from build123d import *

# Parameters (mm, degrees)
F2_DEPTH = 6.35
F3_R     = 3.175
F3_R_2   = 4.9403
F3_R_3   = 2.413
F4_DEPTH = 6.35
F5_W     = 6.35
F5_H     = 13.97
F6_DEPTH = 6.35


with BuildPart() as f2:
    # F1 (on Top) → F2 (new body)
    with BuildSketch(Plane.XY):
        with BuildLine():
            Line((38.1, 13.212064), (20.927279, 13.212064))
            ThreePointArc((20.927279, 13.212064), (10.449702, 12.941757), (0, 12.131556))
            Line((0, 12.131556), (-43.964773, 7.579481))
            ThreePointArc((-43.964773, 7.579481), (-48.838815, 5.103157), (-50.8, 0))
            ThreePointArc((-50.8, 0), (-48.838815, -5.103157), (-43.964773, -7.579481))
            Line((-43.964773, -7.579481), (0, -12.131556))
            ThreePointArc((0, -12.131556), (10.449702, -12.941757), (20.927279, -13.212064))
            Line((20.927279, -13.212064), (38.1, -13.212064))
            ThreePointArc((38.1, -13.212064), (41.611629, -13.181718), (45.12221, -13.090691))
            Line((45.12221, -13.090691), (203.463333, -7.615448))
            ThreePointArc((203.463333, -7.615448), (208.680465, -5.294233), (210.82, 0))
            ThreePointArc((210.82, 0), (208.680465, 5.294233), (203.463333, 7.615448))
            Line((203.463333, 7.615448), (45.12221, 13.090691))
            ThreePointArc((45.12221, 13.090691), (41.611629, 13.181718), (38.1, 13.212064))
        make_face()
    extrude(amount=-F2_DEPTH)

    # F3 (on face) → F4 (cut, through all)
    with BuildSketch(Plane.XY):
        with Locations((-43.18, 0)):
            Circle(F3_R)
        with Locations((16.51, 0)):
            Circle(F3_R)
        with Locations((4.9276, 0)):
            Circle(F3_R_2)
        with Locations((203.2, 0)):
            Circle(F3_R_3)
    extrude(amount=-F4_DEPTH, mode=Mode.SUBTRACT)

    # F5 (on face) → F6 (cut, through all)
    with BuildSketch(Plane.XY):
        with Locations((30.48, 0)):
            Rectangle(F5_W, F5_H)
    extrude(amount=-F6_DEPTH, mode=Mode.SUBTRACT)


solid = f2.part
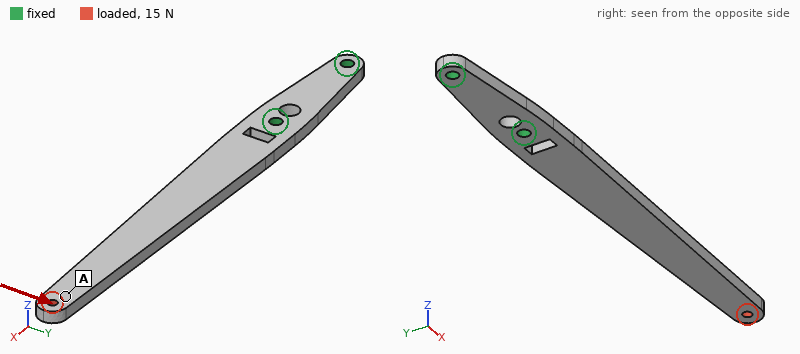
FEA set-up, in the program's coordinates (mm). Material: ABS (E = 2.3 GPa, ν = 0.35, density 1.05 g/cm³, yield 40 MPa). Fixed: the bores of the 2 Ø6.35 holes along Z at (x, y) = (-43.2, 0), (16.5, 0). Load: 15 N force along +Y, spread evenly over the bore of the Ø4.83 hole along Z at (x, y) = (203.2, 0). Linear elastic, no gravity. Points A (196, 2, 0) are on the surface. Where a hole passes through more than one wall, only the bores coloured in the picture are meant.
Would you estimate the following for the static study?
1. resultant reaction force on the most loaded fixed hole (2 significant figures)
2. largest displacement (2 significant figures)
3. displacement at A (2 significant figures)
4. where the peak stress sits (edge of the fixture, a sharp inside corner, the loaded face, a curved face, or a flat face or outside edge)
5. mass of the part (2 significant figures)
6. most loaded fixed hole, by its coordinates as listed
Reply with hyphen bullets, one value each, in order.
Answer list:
- 43 N
- 2.5 mm
- 2.2 mm
- edge of the fixture
- 35 g
- (16.5, 0)
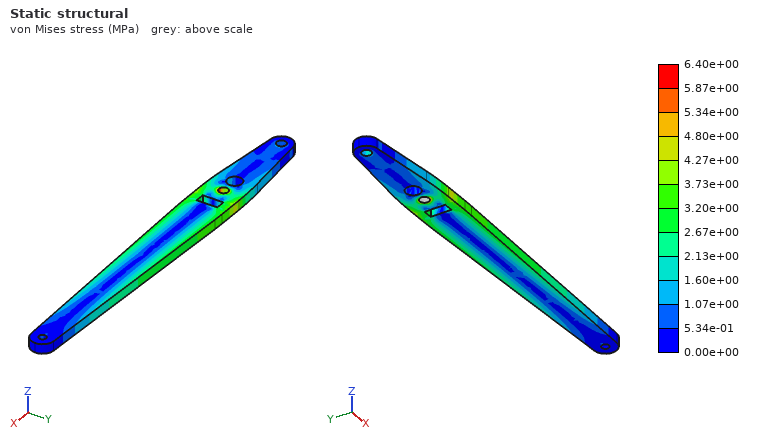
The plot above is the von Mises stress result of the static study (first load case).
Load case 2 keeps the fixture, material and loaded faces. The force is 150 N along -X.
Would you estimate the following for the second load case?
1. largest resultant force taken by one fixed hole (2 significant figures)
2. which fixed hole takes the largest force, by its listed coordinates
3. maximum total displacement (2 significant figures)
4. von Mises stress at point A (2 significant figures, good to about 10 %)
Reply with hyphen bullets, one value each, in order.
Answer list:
- 130 N
- (16.5, 0)
- 0.11 mm
- 1.6 MPa
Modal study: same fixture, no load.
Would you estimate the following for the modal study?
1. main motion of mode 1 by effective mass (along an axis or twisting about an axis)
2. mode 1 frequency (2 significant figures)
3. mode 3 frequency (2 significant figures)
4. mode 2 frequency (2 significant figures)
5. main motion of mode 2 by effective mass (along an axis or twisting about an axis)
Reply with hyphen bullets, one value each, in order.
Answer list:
- along Z
- 44 Hz
- 260 Hz
- 170 Hz
- along Y
